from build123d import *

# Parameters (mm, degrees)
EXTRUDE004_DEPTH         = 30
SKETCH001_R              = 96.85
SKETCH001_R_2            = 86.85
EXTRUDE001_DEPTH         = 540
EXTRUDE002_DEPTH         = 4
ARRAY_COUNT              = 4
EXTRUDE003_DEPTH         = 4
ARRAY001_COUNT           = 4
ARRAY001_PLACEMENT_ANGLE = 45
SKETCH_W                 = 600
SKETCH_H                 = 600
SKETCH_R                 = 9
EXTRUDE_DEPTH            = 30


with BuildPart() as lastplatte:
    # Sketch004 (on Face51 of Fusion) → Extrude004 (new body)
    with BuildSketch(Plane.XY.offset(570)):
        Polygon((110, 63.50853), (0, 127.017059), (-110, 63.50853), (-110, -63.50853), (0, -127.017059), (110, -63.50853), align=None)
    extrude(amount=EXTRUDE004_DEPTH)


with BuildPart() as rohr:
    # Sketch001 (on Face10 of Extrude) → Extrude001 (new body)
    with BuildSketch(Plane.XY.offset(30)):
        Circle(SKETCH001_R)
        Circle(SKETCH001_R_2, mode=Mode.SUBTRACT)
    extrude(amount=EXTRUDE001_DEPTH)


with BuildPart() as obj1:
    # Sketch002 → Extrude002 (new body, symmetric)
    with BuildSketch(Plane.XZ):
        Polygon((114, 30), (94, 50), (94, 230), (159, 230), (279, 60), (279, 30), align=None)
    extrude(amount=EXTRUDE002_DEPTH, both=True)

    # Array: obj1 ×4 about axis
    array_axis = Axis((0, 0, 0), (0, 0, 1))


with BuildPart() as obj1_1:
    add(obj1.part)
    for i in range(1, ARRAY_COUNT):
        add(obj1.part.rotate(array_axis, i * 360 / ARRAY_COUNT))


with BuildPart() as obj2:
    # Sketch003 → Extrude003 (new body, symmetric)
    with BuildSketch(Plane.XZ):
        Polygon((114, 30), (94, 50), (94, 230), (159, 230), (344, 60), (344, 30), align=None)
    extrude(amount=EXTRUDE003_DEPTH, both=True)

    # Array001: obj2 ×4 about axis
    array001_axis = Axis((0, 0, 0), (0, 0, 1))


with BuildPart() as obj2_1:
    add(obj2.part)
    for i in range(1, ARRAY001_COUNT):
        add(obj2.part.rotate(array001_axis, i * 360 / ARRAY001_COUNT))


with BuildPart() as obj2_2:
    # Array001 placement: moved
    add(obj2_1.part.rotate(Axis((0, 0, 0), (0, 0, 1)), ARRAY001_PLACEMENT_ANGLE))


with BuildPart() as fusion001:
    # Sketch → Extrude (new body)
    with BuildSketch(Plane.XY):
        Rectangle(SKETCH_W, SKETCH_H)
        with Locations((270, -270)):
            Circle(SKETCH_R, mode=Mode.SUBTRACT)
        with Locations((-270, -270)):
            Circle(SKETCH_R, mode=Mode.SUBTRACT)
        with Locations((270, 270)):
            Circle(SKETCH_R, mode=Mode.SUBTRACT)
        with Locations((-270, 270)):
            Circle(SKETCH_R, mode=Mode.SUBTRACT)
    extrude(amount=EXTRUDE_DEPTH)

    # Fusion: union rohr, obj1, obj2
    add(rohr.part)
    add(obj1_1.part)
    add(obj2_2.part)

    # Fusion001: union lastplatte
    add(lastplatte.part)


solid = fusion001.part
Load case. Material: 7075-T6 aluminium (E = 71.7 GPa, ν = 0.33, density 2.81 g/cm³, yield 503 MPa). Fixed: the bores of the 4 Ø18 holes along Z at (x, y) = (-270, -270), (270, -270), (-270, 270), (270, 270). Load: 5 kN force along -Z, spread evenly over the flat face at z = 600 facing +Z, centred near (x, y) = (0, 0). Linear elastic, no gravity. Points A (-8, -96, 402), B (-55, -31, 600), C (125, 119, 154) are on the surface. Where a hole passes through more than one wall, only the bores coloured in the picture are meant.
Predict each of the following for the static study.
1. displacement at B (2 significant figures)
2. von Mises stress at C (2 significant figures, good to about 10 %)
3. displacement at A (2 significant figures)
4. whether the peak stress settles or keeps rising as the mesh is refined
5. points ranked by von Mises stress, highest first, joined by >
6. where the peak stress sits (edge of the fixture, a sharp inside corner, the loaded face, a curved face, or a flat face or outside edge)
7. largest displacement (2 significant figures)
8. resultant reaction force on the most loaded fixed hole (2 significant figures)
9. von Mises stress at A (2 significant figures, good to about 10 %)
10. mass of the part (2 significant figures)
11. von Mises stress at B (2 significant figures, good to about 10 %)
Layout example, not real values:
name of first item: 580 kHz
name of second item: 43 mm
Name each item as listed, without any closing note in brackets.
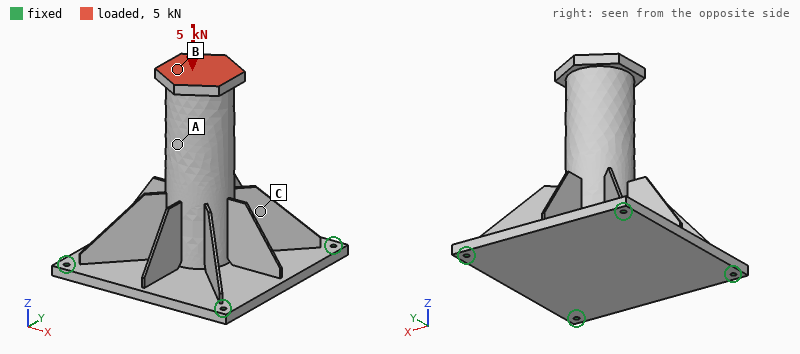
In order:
displacement at B: 27 µm
von Mises stress at C: 1.6 MPa
displacement at A: 24 µm
whether the peak stress settles or keeps rising as the mesh is refined: keeps rising
points ranked by von Mises stress, highest first, joined by >: C > A > B
where the peak stress sits: edge of the fixture
largest displacement: 28 µm
resultant reaction force on the most loaded fixed hole: 1.4 kN
von Mises stress at A: 0.90 MPa
mass of the part: 48 kg
von Mises stress at B: 0.43 MPa
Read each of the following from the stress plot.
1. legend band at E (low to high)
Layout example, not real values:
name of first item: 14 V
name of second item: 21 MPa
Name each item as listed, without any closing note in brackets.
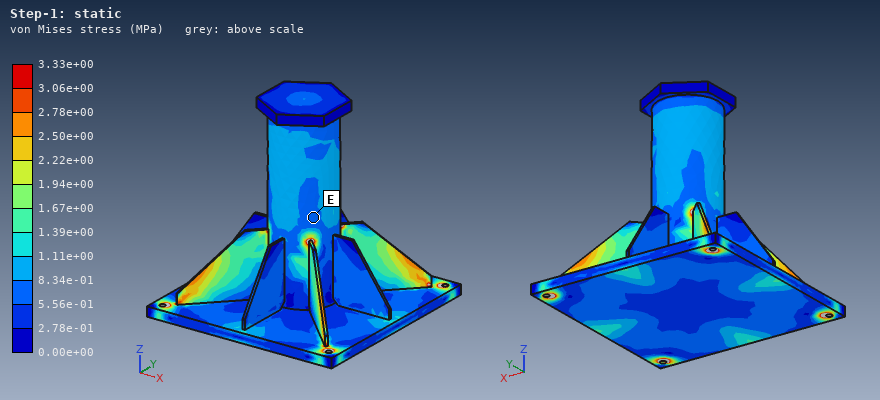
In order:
legend band at E: 5.56e-01 to 8.34e-01 MPa
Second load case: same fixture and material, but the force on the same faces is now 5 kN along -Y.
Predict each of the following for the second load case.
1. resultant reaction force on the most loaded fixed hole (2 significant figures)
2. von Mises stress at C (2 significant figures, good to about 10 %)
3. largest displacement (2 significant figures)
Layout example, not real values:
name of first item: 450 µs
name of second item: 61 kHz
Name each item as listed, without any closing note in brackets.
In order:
resultant reaction force on the most loaded fixed hole: 3.3 kN
von Mises stress at C: 3.7 MPa
largest displacement: 0.25 mm
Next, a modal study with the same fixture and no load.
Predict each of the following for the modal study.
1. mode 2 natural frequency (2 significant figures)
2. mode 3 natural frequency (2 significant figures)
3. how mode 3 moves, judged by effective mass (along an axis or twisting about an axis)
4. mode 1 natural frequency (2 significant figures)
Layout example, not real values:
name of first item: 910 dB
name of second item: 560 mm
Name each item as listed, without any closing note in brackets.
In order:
mode 2 natural frequency: 300 Hz
mode 3 natural frequency: 400 Hz
how mode 3 moves, judged by effective mass: along Z
mode 1 natural frequency: 300 Hz
